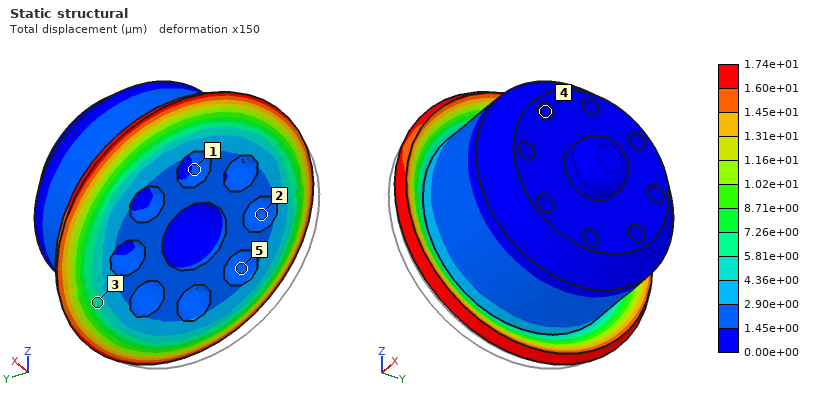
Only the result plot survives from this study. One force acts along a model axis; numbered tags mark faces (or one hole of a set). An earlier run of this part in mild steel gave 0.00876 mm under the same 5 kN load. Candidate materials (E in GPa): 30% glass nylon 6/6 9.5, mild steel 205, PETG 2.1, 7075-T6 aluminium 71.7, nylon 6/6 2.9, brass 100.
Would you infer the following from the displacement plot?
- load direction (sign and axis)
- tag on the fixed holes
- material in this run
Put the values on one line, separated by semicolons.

+X; 4; brass
